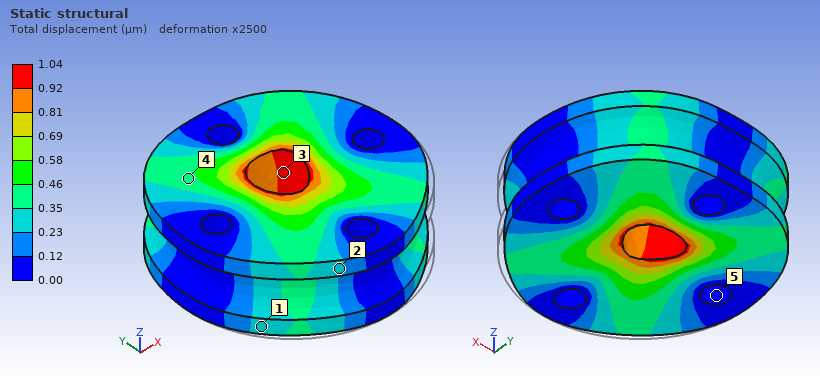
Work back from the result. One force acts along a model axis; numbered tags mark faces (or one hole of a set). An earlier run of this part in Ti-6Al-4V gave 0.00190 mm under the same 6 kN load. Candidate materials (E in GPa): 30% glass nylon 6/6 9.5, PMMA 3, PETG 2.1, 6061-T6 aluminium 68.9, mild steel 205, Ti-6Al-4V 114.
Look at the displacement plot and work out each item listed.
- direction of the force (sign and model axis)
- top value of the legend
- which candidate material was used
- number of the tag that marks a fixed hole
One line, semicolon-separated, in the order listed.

+Y; 1.04 µm; mild steel; 5
